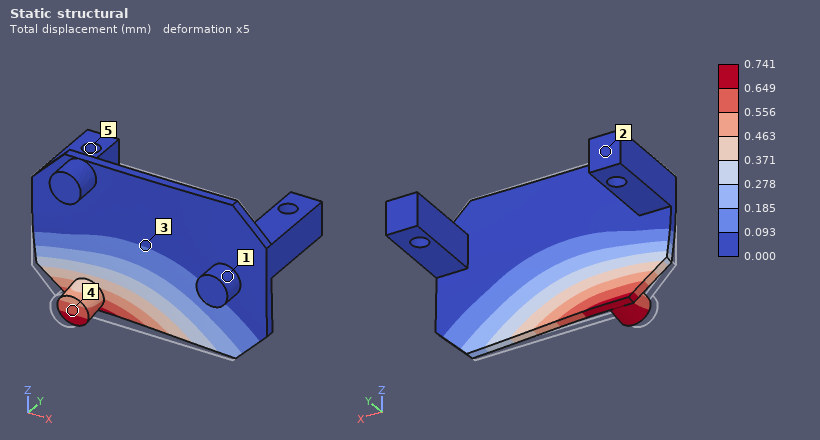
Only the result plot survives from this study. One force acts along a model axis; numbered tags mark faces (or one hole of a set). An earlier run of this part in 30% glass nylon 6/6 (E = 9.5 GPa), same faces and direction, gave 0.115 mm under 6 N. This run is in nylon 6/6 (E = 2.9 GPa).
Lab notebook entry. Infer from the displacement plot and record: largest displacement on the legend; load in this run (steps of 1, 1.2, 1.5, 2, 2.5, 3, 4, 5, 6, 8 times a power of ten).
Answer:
0.741 mm
12 N
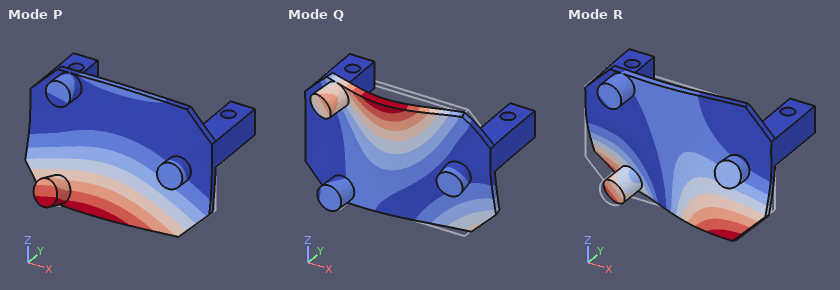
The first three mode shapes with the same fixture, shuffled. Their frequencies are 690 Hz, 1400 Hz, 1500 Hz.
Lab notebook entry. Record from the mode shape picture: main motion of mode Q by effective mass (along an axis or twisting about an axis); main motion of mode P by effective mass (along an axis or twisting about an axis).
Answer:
along Y
along Y
